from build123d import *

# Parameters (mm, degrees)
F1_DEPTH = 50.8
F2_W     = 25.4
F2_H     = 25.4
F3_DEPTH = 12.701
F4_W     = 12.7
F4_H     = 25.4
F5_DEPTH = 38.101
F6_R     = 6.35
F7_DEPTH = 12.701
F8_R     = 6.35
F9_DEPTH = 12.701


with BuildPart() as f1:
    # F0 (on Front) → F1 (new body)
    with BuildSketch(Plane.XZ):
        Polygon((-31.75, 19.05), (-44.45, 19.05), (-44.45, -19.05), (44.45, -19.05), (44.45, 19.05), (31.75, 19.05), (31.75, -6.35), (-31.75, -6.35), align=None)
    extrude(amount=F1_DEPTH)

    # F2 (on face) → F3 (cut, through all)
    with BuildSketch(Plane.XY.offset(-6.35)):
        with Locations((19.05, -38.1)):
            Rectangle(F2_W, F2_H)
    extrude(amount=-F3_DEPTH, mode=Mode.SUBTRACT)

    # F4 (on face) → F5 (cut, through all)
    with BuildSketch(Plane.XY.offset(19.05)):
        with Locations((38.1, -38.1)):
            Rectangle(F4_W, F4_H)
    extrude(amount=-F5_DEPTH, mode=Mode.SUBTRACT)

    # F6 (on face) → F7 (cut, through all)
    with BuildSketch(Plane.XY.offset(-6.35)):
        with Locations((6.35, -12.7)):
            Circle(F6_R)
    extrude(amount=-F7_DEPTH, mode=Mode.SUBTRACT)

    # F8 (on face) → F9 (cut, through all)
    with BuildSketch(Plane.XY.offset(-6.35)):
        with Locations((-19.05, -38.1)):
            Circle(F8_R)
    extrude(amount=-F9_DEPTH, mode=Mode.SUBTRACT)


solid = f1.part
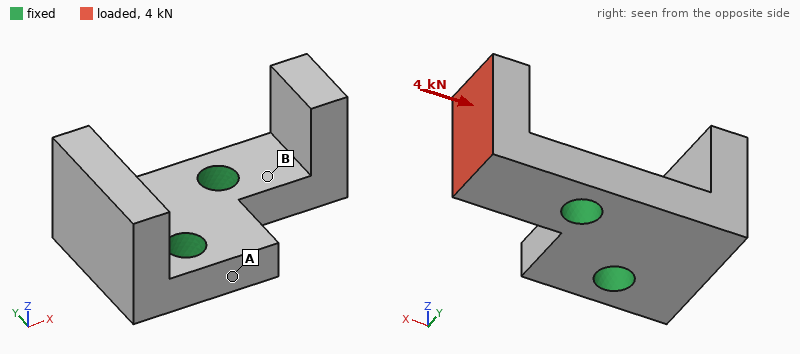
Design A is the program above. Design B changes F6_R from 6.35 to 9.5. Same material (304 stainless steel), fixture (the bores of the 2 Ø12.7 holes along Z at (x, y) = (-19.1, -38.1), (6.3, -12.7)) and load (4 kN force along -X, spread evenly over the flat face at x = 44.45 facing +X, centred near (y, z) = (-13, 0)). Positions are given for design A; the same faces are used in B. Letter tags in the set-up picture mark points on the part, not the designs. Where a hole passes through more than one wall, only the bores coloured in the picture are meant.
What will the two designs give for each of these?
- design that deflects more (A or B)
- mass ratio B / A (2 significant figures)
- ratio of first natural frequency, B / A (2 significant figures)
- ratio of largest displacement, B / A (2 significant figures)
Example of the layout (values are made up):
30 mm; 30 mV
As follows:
A; 0.97; 1.1; 0.86
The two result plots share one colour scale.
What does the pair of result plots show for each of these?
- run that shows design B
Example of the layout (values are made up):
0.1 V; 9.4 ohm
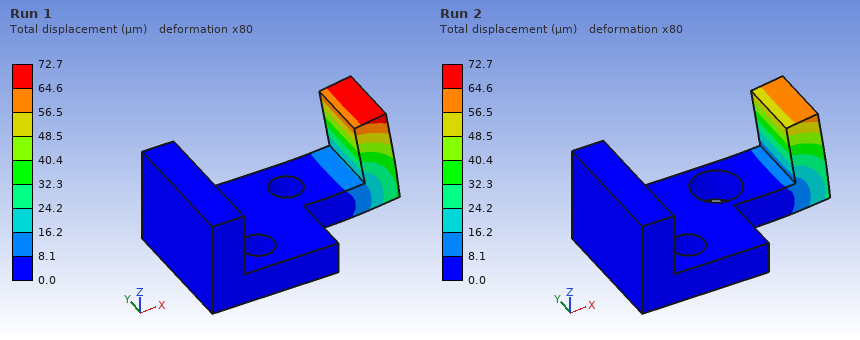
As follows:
Run 2
